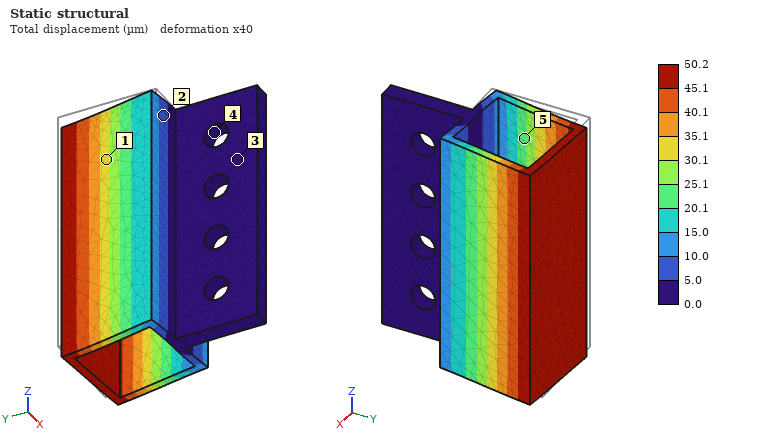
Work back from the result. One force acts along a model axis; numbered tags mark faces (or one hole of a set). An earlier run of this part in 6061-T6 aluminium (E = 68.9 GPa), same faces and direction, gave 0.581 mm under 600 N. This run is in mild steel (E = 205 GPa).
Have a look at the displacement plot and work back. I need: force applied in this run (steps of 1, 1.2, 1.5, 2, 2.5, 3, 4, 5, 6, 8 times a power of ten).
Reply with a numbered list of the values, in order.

1. 150 N
